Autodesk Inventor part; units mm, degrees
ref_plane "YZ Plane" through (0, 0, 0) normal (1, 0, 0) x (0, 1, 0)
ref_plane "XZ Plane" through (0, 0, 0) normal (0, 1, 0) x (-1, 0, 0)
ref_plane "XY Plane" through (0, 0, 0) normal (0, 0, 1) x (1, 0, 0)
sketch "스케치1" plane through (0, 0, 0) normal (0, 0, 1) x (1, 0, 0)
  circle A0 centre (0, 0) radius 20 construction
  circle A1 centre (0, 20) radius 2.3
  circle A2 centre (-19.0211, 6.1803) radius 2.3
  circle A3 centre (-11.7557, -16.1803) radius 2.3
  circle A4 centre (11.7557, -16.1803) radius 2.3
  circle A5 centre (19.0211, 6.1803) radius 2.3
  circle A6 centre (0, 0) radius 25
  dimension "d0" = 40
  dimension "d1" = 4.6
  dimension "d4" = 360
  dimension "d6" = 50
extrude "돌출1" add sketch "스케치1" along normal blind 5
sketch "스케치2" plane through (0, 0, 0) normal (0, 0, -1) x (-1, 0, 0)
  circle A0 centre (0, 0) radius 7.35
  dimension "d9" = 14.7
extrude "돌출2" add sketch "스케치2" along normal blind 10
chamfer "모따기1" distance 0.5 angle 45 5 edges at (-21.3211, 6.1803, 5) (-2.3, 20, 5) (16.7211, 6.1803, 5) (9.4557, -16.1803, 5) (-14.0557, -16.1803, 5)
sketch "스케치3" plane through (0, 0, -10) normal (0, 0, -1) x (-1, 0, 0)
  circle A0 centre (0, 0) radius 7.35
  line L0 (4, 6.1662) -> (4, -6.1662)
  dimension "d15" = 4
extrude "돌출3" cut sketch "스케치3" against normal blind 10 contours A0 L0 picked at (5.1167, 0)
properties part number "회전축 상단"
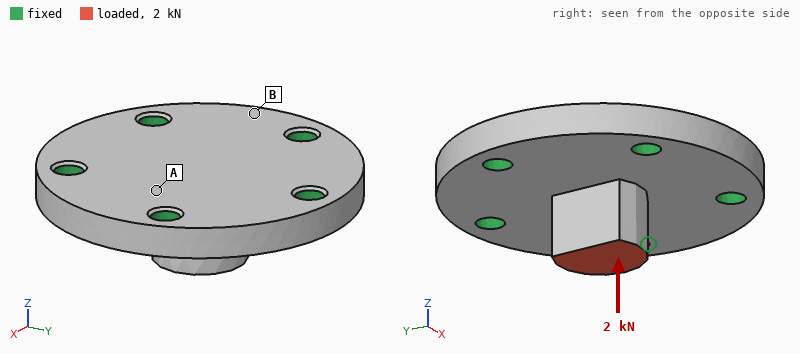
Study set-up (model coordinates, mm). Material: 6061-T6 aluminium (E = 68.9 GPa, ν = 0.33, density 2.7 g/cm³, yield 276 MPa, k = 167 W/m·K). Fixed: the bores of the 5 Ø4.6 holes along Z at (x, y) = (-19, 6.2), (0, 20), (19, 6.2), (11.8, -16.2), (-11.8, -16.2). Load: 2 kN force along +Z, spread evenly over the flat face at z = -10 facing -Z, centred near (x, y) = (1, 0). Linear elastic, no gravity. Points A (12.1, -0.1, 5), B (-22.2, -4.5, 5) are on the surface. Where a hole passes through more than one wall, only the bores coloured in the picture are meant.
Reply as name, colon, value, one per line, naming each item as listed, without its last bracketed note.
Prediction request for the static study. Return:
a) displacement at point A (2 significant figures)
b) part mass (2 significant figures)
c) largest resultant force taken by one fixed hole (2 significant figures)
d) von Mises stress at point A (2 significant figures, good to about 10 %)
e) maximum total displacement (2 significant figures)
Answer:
displacement at point A: 7.6 µm
part mass: 29 g
largest resultant force taken by one fixed hole: 440 N
von Mises stress at point A: 15 MPa
maximum total displacement: 16 µm
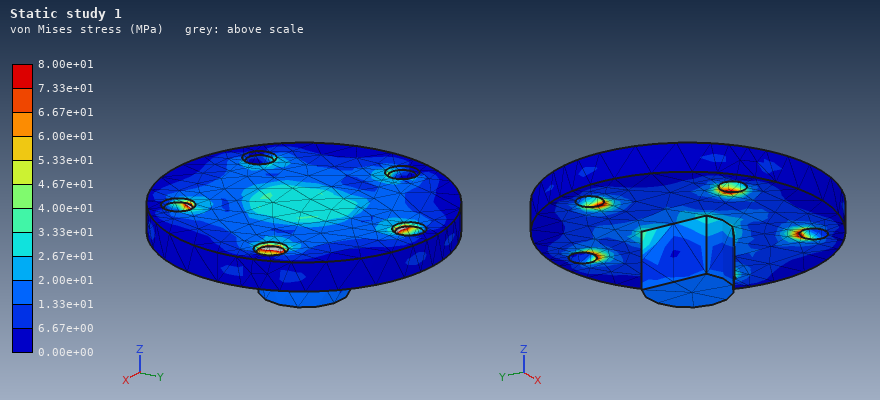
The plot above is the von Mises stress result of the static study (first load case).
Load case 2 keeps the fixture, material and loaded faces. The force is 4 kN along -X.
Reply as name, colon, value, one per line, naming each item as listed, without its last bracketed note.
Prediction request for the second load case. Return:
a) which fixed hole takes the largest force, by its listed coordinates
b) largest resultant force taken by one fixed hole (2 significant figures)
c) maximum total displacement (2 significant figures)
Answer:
which fixed hole takes the largest force, by its listed coordinates: (19, 6.2)
largest resultant force taken by one fixed hole: 1.8 kN
maximum total displacement: 87 µm
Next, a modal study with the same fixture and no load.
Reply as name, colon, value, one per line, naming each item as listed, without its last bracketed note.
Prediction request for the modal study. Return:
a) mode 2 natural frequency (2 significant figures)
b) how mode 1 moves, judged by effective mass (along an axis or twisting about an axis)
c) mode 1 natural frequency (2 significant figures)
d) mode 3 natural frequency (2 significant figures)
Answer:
mode 2 natural frequency: 26 kHz
how mode 1 moves, judged by effective mass: along Z
mode 1 natural frequency: 20 kHz
mode 3 natural frequency: 27 kHz
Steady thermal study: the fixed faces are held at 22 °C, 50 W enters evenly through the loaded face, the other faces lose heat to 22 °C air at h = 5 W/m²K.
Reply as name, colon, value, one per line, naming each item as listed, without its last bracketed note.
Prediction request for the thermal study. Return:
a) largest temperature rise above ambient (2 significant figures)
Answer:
largest temperature rise above ambient: 37 K
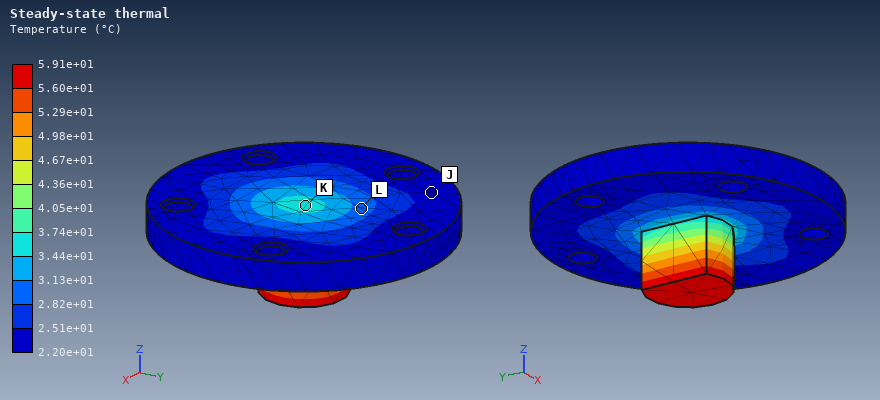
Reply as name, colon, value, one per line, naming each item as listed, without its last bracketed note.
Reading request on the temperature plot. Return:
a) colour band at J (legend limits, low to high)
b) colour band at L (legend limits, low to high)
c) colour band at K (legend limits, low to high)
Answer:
colour band at J: 2.20e+01 to 2.51e+01 °C
colour band at L: 2.82e+01 to 3.13e+01 °C
colour band at K: 3.44e+01 to 3.74e+01 °C
